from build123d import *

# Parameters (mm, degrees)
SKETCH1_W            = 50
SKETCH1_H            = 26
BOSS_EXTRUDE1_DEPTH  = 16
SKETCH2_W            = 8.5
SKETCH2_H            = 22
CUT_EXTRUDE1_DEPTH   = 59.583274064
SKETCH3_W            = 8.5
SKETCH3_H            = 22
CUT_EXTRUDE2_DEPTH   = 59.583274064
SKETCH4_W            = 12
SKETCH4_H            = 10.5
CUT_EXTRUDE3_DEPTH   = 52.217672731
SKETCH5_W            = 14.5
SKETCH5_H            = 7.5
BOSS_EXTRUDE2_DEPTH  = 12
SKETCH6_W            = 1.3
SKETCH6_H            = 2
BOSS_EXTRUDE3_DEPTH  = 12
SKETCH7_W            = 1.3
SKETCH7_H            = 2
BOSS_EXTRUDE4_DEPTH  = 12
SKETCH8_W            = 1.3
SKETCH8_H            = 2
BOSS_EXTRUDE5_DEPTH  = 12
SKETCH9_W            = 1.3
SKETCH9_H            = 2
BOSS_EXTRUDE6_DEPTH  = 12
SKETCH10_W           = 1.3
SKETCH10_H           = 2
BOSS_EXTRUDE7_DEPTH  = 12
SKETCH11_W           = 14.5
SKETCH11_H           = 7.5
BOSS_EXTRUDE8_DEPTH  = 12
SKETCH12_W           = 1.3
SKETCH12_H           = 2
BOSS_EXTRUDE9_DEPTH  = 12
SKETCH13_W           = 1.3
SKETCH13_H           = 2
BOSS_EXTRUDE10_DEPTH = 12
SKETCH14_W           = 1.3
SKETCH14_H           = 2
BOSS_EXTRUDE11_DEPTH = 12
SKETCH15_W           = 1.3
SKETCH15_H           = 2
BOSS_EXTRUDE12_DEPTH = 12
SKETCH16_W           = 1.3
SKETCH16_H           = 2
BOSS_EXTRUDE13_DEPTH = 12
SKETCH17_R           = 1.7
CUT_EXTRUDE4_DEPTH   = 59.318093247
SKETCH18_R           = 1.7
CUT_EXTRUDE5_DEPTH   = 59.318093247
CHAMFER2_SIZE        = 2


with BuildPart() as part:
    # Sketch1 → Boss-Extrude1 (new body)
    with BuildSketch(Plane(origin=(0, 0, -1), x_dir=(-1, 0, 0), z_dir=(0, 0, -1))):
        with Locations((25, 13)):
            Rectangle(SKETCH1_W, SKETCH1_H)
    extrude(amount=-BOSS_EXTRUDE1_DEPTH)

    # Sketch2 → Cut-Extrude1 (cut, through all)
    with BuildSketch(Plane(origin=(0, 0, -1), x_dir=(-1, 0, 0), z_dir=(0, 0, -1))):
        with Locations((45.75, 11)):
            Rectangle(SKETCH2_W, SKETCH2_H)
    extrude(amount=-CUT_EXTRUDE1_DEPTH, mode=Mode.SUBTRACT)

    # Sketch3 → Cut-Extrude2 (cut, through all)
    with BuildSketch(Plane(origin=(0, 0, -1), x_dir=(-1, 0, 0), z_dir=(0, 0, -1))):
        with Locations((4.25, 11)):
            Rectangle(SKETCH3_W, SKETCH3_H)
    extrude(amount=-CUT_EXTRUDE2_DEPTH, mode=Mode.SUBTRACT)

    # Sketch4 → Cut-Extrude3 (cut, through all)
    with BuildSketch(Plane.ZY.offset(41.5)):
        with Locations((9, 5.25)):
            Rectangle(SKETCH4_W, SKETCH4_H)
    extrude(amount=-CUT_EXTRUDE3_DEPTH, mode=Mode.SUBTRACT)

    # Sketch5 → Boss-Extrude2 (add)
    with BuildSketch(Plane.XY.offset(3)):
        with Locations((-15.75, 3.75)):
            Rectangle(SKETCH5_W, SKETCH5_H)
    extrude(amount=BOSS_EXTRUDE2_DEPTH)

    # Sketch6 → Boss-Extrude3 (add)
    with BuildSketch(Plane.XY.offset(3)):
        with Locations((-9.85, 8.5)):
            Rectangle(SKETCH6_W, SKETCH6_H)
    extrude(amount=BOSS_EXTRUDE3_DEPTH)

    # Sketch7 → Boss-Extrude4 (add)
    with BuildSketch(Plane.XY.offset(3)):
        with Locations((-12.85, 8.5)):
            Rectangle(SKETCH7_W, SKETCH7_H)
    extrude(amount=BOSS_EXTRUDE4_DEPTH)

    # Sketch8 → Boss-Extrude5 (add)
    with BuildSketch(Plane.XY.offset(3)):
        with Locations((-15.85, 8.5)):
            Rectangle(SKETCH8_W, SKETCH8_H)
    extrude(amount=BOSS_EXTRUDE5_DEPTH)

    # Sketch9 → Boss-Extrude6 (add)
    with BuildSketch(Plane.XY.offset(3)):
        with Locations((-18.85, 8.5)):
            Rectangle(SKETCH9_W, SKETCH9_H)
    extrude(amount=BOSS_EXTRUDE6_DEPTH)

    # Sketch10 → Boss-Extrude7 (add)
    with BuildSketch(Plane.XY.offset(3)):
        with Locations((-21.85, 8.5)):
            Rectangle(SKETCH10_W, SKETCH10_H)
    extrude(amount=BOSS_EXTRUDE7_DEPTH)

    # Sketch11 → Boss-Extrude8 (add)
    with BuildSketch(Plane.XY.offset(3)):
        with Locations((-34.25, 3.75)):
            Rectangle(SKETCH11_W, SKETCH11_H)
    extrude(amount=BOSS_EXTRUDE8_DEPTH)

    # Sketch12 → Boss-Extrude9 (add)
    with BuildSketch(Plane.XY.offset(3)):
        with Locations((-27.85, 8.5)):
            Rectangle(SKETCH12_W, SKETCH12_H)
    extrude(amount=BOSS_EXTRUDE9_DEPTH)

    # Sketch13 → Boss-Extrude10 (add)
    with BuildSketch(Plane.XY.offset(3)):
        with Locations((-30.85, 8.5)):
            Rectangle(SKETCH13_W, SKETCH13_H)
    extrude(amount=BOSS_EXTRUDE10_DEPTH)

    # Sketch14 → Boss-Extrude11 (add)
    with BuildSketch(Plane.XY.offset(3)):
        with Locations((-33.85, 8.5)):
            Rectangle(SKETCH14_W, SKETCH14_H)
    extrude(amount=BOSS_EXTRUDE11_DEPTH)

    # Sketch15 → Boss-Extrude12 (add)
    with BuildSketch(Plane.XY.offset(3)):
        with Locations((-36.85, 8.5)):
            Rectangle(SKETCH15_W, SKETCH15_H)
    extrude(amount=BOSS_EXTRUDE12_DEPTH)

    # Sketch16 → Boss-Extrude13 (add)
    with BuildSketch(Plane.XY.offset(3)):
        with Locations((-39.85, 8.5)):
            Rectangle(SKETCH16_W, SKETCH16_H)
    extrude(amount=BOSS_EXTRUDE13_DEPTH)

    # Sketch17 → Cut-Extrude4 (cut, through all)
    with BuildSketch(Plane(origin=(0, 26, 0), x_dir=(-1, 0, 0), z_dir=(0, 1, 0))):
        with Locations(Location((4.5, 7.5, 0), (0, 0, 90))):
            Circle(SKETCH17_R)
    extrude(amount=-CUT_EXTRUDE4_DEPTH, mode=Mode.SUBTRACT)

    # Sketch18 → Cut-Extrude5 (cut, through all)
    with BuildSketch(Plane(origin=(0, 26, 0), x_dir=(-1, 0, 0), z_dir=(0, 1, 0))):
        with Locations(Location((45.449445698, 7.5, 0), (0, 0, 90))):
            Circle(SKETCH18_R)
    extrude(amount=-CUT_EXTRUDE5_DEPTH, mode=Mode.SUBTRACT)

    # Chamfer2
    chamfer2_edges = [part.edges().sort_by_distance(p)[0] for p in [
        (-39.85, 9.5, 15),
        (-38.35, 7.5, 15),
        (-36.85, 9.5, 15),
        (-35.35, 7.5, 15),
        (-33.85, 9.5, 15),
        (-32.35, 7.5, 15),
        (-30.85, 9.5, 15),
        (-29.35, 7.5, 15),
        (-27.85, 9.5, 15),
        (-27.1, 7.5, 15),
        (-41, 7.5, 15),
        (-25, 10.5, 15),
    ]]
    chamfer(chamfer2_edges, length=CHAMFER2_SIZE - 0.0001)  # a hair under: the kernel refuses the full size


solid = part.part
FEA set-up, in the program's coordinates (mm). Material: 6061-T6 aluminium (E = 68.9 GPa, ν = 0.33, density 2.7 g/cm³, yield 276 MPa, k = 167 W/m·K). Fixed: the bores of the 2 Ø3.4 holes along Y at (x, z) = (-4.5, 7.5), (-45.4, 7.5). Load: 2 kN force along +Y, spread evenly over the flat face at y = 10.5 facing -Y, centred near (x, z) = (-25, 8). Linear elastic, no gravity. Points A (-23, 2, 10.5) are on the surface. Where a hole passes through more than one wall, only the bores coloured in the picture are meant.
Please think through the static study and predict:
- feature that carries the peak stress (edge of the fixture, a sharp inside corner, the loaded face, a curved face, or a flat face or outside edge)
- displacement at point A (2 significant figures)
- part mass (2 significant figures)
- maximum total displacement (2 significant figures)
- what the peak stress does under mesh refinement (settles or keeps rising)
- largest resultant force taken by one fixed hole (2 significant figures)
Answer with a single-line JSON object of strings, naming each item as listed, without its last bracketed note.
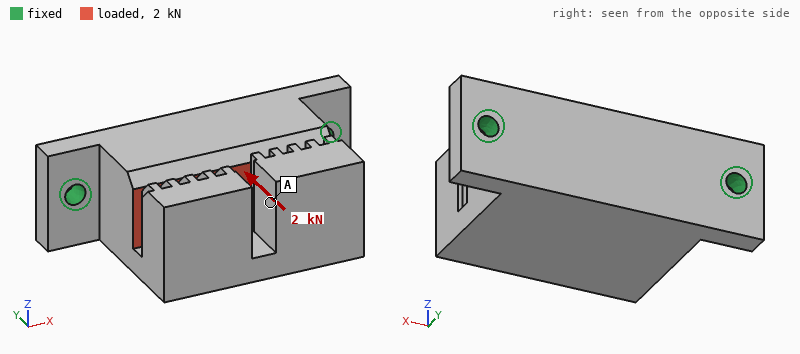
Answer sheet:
{"feature that carries the peak stress": "edge of the fixture", "displacement at point A": "14 µm", "part mass": "36 g", "maximum total displacement": "17 µm", "what the peak stress does under mesh refinement": "keeps rising", "largest resultant force taken by one fixed hole": "1.1 kN"}
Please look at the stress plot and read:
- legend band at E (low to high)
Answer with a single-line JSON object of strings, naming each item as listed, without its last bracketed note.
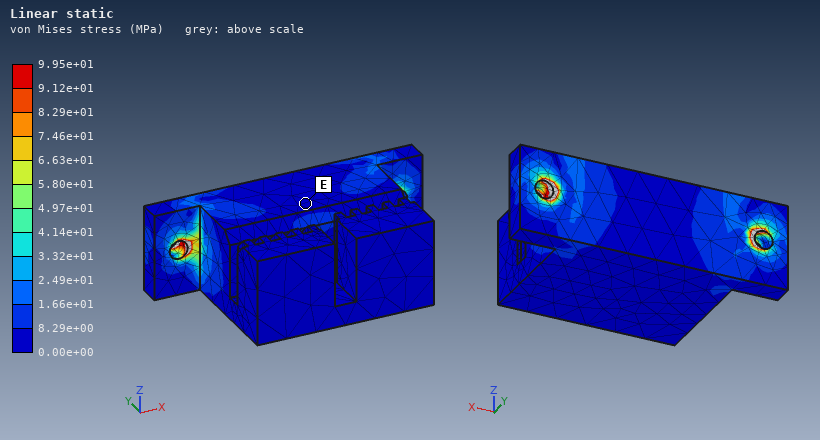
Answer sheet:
{"legend band at E": "0.00e+00 to 8.29e+00 MPa"}
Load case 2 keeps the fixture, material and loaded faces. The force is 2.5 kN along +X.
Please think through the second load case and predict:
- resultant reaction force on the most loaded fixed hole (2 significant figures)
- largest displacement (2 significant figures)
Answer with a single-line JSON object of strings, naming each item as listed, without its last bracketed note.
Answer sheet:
{"resultant reaction force on the most loaded fixed hole": "1.6 kN", "largest displacement": "16 µm"}
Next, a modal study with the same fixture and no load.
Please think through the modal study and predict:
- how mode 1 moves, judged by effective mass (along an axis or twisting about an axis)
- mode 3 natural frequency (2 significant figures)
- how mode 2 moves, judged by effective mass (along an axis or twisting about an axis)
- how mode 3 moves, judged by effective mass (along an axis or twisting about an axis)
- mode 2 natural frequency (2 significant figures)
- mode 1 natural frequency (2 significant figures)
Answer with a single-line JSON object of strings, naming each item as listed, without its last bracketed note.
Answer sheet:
{"how mode 1 moves, judged by effective mass": "along Z", "mode 3 natural frequency": "9800 Hz", "how mode 2 moves, judged by effective mass": "along Y", "how mode 3 moves, judged by effective mass": "along X", "mode 2 natural frequency": "8700 Hz", "mode 1 natural frequency": "3400 Hz"}
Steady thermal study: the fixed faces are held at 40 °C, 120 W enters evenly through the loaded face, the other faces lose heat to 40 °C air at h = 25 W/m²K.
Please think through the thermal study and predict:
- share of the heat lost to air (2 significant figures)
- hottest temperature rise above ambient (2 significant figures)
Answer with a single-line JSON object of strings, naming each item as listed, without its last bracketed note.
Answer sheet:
{"share of the heat lost to air": "4.9 %", "hottest temperature rise above ambient": "64 K"}
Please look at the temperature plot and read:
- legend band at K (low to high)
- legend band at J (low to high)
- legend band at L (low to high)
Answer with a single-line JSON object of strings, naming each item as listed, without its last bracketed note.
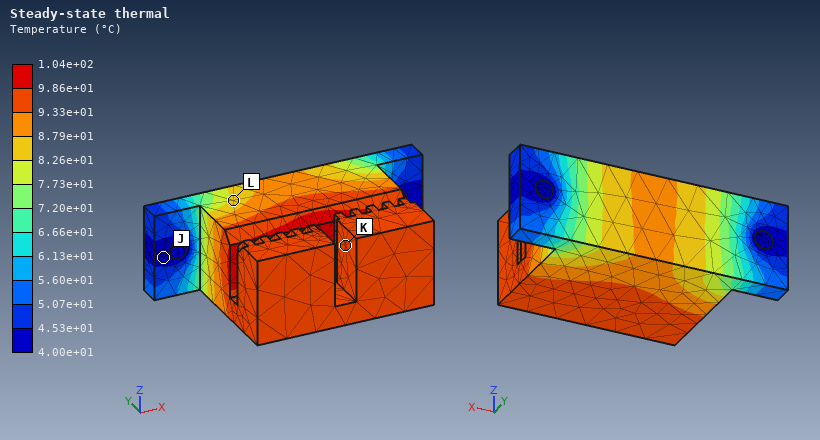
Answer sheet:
{"legend band at K": "9.33e+01 to 9.86e+01 °C", "legend band at J": "4.00e+01 to 4.53e+01 °C", "legend band at L": "8.26e+01 to 8.79e+01 °C"}
